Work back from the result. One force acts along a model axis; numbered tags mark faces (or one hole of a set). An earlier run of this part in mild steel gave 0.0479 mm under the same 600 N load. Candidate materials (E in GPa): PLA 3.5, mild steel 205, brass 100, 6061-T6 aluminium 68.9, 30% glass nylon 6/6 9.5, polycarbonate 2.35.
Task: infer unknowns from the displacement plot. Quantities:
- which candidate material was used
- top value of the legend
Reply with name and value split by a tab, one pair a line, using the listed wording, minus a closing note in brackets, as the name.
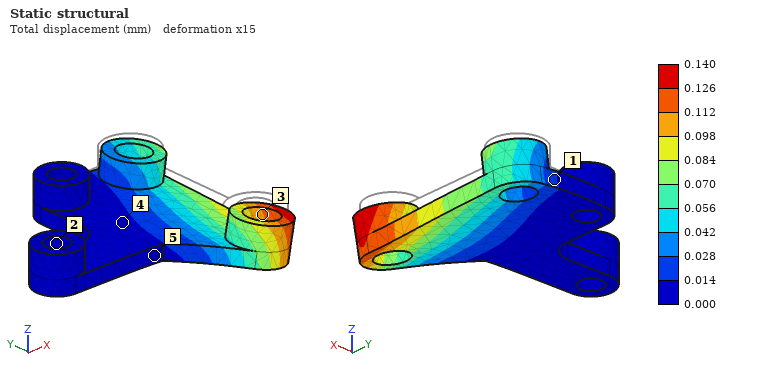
which candidate material was used	6061-T6 aluminium
top value of the legend	0.140 mm
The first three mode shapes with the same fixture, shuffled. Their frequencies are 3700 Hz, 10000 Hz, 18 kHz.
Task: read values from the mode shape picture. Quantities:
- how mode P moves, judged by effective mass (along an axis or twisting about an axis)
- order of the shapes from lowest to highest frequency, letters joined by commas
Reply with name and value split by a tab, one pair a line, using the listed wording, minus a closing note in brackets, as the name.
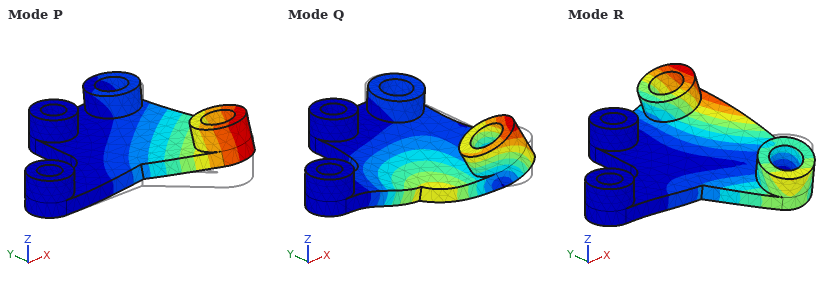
how mode P moves, judged by effective mass	along Z
order of the shapes from lowest to highest frequency, letters joined by commas	P, R, Q
